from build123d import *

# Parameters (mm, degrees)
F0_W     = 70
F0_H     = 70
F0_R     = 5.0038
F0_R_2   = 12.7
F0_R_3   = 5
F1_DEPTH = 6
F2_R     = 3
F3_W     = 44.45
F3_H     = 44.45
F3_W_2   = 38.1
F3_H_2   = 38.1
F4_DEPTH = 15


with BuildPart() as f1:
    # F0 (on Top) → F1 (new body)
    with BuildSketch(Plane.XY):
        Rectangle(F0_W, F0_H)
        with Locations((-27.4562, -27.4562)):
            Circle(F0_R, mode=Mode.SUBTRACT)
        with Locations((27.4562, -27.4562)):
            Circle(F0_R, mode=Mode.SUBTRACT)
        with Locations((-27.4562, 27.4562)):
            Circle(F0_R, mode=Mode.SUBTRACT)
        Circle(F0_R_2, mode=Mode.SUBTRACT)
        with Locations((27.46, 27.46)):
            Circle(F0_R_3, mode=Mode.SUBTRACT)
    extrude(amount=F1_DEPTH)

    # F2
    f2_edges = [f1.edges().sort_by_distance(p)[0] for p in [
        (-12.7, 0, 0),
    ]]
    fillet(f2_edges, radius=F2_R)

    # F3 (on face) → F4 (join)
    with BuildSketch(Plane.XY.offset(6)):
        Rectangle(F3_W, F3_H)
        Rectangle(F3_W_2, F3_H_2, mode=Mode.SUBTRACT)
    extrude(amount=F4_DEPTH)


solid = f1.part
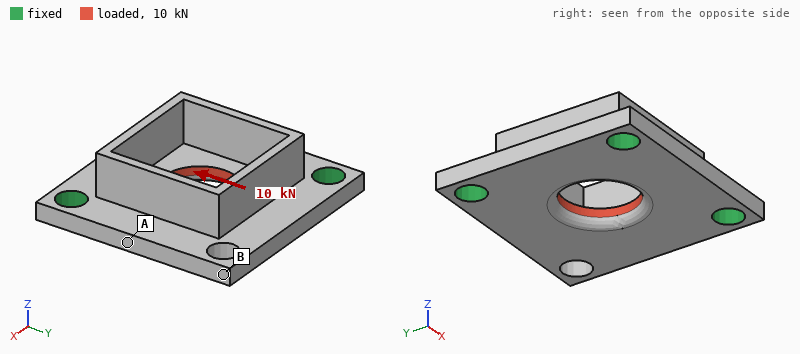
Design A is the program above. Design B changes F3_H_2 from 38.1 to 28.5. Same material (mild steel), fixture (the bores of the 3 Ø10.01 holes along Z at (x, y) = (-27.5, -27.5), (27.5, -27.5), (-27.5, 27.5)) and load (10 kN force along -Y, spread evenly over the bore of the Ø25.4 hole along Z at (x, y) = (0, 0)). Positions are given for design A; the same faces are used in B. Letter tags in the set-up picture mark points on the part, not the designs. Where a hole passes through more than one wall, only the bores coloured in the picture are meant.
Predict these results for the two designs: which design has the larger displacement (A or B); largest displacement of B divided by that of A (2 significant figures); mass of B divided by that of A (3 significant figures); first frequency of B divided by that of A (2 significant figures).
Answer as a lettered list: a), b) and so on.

a) A
b) 0.74
c) 1.17
d) 1.1
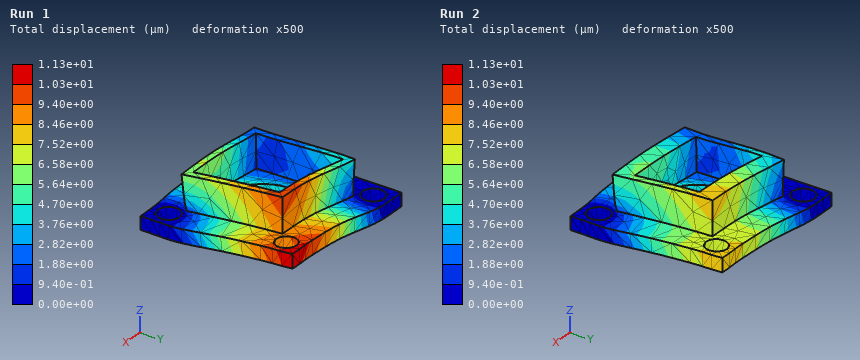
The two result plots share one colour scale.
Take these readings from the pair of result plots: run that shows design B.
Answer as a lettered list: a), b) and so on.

a) Run 2
